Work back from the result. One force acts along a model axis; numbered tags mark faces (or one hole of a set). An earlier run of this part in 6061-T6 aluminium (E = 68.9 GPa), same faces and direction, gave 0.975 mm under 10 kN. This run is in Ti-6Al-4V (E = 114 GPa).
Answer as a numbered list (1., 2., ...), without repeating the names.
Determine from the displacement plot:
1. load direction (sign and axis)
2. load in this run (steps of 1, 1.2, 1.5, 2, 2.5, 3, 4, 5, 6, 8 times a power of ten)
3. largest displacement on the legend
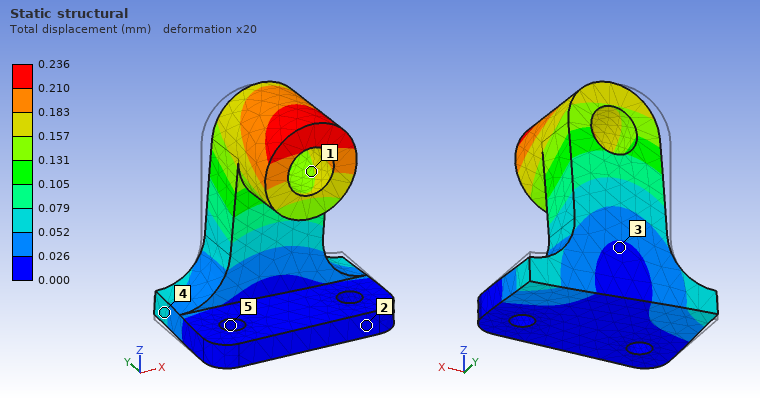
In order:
1. +X
2. 4 kN
3. 0.236 mm
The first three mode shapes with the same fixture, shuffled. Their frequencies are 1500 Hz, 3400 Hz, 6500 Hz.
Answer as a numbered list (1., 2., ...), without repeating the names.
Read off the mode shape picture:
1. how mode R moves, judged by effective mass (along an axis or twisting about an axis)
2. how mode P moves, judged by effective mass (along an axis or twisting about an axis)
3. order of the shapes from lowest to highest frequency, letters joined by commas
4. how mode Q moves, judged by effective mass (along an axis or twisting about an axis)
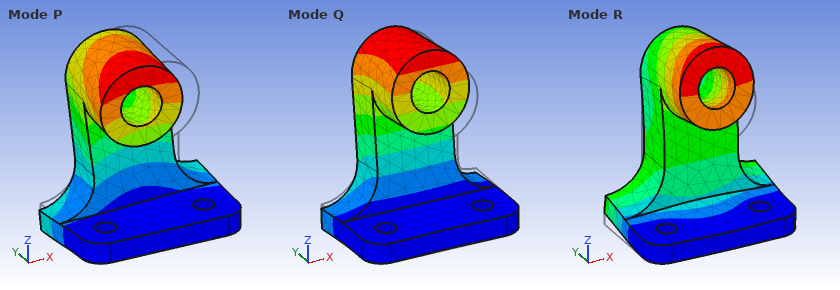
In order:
1. along Z
2. along X
3. Q, P, R
4. along Y
